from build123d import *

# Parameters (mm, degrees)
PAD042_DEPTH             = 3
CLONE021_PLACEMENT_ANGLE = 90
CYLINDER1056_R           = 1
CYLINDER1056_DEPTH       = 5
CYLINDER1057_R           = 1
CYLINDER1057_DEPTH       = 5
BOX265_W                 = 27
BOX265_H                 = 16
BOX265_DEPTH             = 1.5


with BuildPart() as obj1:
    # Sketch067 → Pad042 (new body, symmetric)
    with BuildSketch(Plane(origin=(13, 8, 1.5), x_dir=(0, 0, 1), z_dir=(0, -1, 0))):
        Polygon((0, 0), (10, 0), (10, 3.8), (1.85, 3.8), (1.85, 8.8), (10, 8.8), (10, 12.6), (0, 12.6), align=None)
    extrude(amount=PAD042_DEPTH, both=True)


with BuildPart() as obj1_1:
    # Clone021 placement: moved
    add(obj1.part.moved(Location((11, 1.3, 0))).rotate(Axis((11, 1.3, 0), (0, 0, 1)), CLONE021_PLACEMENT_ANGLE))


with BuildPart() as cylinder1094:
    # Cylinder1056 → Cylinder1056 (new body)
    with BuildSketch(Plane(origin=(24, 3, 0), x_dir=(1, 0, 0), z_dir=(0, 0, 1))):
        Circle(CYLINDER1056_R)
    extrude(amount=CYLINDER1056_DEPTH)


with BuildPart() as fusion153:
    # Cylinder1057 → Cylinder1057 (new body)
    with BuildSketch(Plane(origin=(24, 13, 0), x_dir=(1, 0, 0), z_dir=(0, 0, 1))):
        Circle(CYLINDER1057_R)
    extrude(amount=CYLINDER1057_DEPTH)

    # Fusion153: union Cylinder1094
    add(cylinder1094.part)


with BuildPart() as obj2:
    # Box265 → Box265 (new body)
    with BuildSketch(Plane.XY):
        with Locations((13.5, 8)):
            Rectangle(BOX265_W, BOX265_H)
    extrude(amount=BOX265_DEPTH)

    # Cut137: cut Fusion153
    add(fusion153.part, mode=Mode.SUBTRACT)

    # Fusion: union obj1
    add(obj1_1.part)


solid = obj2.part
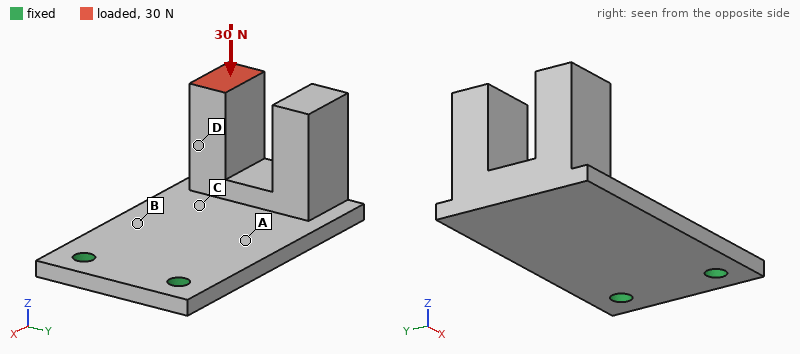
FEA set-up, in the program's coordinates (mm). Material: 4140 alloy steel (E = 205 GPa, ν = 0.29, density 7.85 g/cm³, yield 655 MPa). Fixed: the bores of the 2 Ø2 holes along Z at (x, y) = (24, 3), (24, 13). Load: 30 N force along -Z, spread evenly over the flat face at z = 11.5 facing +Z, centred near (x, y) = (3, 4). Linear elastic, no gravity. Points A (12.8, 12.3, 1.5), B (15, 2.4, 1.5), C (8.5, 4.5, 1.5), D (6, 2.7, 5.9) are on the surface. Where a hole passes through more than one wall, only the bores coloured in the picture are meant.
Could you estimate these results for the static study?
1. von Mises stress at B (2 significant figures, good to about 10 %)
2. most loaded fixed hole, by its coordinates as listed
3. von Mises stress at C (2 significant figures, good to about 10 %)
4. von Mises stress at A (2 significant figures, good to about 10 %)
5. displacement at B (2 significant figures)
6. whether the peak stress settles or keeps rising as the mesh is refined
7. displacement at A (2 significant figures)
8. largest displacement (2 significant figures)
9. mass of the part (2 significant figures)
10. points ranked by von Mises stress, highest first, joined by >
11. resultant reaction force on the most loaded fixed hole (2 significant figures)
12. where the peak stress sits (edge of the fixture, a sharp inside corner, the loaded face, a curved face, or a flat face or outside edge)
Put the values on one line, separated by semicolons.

63 MPa; (24, 3); 28 MPa; 49 MPa; 0.025 mm; keeps rising; 0.030 mm; 0.14 mm; 9.0 g; B > A > C > D; 26 N; edge of the fixture
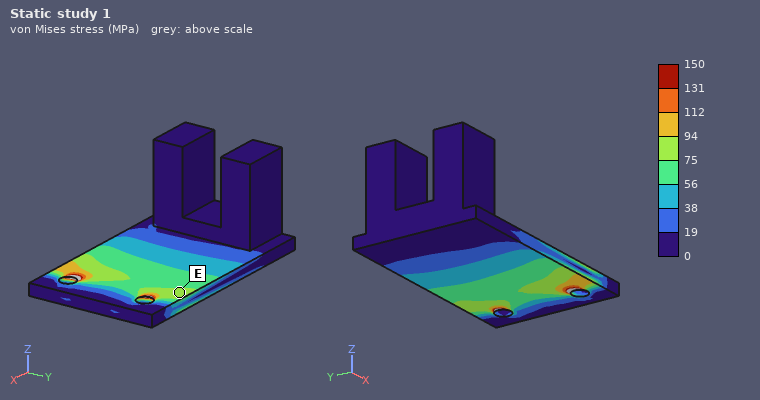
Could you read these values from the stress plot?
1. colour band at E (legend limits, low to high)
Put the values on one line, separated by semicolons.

75 to 94 MPa
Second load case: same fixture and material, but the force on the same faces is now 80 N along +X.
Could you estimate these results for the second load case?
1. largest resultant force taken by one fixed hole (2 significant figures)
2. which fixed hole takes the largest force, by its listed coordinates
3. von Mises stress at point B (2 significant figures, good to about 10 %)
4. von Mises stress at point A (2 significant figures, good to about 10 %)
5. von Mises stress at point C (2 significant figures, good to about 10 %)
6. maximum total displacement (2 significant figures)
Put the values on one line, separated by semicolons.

73 N; (24, 3); 150 MPa; 140 MPa; 140 MPa; 0.31 mm
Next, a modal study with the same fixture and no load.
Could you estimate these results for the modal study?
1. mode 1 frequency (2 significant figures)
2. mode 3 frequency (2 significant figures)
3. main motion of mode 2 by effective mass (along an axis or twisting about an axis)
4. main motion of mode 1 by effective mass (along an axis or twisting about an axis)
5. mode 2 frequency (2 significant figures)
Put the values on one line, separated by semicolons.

1100 Hz; 6100 Hz; along Y; along Z; 3200 Hz
